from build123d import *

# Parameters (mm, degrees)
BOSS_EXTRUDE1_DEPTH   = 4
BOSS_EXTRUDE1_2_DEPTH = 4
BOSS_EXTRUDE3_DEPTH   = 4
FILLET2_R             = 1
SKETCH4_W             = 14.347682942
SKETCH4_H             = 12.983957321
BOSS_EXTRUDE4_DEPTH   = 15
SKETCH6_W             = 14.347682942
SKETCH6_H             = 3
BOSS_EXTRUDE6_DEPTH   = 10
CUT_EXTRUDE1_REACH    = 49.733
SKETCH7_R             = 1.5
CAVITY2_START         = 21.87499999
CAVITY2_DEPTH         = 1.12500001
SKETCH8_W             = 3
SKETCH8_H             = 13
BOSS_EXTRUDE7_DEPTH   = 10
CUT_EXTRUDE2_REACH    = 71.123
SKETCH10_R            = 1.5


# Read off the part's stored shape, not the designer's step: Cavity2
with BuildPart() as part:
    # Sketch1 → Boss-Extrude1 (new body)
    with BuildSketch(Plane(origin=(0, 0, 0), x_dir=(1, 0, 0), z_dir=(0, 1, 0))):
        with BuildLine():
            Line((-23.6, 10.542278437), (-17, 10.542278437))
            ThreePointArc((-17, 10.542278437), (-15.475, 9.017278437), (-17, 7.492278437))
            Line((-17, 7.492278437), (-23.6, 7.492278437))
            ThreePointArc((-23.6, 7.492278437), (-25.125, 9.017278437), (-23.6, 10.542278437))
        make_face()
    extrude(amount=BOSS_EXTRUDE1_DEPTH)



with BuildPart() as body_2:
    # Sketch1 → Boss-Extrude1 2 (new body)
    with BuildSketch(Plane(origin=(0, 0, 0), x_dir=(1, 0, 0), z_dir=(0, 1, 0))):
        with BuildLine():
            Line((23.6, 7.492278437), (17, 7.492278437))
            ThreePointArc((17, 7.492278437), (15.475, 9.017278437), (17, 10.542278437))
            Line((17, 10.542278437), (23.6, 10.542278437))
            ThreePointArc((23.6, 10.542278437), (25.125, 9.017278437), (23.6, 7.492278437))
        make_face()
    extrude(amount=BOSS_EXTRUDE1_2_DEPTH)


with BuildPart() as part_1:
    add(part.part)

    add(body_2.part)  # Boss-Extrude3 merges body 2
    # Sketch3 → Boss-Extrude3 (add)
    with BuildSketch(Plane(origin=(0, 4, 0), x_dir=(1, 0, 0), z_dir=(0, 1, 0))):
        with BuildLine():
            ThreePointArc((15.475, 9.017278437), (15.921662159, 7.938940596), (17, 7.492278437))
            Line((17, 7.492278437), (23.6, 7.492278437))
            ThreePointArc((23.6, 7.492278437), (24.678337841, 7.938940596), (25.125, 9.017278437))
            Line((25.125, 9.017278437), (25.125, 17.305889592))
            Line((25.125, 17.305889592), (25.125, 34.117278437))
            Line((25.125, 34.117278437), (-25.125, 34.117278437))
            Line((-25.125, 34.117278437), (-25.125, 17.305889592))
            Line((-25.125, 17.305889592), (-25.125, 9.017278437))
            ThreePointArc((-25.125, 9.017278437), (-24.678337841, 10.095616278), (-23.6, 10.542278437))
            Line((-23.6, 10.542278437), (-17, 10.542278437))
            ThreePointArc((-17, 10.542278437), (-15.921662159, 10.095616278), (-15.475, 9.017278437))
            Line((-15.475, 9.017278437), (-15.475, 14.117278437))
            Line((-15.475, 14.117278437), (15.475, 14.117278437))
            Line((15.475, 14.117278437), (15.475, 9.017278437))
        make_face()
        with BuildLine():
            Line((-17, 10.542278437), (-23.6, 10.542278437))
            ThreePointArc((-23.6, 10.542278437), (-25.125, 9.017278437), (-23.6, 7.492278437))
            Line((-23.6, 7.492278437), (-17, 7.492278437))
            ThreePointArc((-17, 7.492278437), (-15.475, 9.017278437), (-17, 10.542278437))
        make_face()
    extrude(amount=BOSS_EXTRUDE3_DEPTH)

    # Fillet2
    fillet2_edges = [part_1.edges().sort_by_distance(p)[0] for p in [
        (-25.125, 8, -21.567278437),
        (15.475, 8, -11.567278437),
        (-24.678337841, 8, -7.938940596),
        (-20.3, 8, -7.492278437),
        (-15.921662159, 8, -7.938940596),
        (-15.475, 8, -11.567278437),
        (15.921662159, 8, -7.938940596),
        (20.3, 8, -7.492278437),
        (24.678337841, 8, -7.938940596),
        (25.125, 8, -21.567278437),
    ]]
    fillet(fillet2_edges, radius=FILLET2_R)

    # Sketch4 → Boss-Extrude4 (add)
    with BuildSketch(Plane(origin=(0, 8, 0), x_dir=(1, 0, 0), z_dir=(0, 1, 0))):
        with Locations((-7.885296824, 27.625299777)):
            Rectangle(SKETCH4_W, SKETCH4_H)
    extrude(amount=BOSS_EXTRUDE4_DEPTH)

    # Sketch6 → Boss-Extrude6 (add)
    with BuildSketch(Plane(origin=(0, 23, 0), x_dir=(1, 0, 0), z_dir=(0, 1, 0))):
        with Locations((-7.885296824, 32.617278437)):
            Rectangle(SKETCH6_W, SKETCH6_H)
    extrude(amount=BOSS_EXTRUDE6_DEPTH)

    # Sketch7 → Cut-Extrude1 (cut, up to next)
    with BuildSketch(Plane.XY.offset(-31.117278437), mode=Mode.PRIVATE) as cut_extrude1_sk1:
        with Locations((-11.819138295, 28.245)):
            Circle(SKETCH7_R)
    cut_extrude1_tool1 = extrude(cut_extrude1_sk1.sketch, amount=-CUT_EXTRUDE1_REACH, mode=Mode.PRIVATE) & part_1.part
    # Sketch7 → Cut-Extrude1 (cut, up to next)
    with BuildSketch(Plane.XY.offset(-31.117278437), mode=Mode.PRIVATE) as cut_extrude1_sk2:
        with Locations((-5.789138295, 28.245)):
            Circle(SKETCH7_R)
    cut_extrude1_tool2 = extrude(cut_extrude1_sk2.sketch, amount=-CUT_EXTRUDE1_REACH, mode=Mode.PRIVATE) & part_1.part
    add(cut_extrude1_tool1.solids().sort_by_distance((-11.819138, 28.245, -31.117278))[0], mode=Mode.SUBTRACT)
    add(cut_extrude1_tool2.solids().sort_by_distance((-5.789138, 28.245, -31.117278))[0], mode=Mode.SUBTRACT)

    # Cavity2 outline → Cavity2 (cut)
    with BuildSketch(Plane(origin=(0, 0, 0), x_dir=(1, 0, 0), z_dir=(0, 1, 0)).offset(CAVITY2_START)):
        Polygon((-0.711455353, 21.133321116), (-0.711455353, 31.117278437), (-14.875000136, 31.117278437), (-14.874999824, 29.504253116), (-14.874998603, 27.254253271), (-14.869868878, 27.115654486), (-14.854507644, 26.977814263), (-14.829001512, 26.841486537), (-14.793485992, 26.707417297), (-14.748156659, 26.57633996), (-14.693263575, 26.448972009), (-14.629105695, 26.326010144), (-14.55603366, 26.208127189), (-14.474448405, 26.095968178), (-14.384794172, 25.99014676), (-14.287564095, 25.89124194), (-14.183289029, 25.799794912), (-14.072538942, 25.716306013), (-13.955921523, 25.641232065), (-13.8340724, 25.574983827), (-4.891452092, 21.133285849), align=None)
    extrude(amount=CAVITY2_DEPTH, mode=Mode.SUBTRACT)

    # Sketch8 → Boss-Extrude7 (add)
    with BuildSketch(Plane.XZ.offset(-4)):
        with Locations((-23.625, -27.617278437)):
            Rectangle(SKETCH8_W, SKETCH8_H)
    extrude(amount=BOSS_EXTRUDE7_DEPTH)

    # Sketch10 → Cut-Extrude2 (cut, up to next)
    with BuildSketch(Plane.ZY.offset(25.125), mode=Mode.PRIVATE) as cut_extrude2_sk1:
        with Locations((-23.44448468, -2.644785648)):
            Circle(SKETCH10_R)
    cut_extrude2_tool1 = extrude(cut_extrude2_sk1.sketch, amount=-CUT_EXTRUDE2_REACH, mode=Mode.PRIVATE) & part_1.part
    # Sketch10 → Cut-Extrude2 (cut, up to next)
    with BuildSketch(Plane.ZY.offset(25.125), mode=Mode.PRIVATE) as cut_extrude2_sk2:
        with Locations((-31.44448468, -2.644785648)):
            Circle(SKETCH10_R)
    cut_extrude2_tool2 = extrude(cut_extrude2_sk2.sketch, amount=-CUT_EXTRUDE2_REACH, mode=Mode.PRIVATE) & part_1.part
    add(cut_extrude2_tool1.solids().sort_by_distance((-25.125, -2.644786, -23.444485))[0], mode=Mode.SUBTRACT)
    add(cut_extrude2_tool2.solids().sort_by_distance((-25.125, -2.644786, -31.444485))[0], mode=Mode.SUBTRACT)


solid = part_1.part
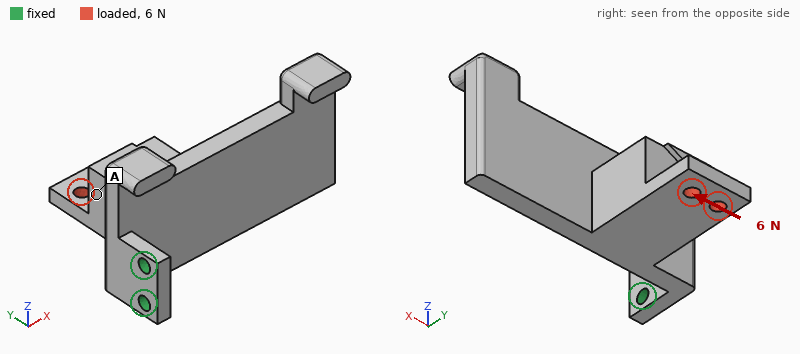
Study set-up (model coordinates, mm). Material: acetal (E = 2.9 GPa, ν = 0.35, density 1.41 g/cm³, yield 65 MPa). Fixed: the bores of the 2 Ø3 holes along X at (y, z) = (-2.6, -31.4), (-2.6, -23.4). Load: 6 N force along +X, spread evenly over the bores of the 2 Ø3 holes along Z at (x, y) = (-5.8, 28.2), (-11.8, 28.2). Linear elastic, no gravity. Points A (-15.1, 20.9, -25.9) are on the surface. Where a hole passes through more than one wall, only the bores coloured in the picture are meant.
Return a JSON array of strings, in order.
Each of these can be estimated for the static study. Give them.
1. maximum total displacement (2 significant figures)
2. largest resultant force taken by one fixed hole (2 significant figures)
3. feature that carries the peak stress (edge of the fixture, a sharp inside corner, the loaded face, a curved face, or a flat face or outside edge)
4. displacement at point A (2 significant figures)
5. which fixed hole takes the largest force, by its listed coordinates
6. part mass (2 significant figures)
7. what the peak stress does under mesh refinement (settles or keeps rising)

["0.82 mm", "6.4 N", "edge of the fixture", "0.34 mm", "(-2.6, -31.4)", "11 g", "keeps rising"]
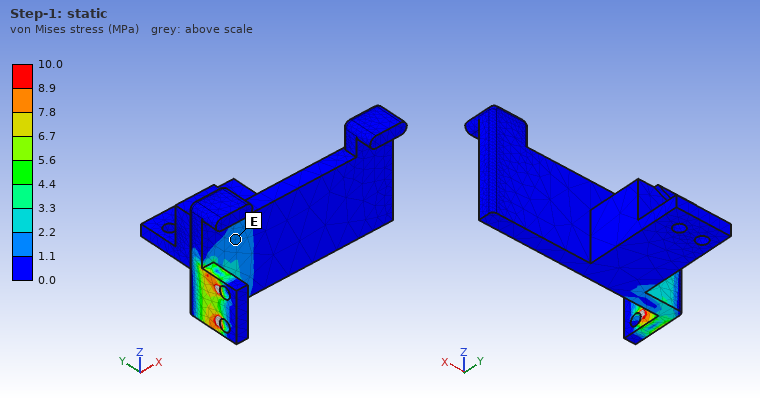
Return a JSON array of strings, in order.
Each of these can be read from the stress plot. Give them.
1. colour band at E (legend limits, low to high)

["1.1 to 2.2 MPa"]
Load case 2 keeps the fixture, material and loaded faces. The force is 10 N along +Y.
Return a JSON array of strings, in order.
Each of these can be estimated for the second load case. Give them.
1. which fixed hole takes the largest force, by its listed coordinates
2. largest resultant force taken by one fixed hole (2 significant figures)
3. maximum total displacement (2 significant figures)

["(-2.6, -31.4)", "11 N", "0.72 mm"]
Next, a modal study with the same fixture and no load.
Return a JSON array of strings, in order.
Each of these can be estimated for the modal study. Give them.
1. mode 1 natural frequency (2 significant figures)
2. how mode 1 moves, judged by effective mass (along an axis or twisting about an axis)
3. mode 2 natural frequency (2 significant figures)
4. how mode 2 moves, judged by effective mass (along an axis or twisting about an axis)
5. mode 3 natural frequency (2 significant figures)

["180 Hz", "along Y", "350 Hz", "along Z", "910 Hz"]
